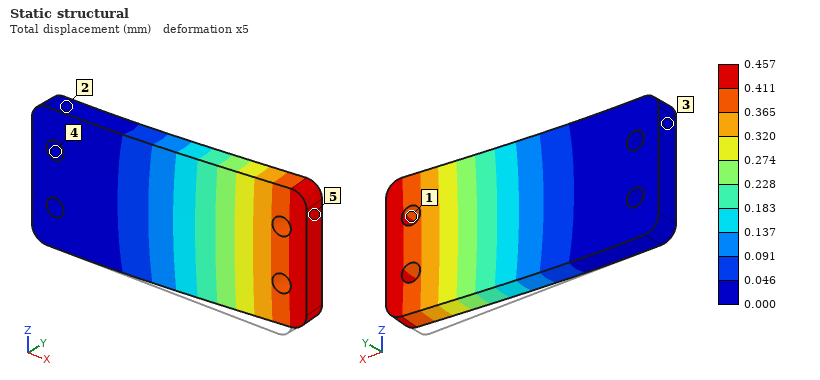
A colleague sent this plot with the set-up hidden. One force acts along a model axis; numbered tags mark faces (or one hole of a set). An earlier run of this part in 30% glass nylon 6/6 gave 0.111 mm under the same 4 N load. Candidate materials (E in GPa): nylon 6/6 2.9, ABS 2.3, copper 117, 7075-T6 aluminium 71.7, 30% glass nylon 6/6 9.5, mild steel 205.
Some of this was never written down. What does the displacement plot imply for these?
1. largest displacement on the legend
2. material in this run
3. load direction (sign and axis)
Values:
0.457 mm
ABS
+Y
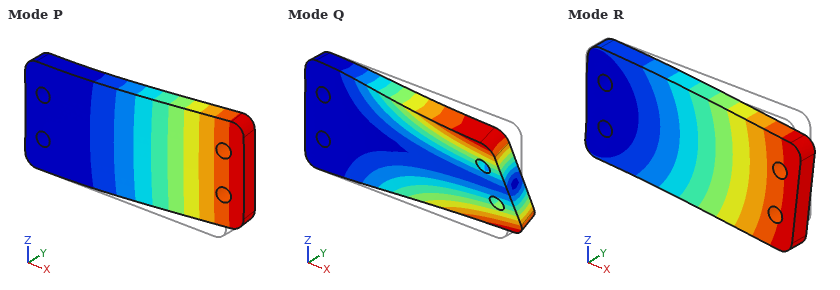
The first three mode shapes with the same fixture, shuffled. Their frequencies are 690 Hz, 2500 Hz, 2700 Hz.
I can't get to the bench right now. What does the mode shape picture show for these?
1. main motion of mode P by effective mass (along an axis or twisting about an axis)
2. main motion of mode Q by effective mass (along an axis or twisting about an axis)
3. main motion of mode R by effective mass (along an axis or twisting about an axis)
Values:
along Y
twisting about X
along Z
